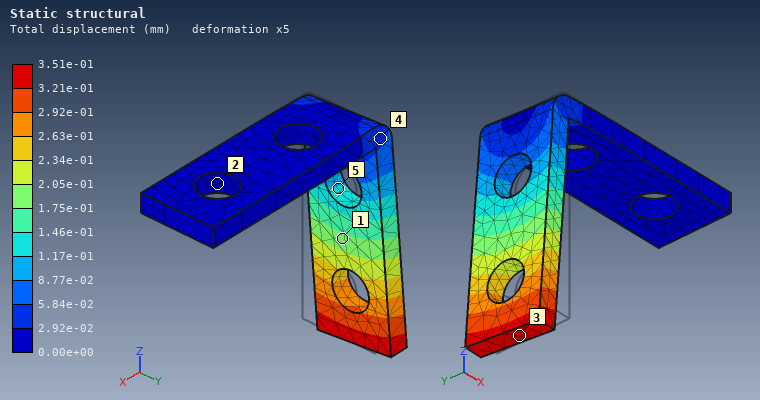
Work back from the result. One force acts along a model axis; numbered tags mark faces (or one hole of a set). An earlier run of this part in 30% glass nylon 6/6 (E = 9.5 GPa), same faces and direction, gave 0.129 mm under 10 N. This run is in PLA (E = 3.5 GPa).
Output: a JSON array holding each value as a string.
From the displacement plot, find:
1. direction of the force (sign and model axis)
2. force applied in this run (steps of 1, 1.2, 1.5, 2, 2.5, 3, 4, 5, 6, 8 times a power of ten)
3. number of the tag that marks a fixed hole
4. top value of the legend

["+Y", "10 N", "2", "3.51e-01 mm"]
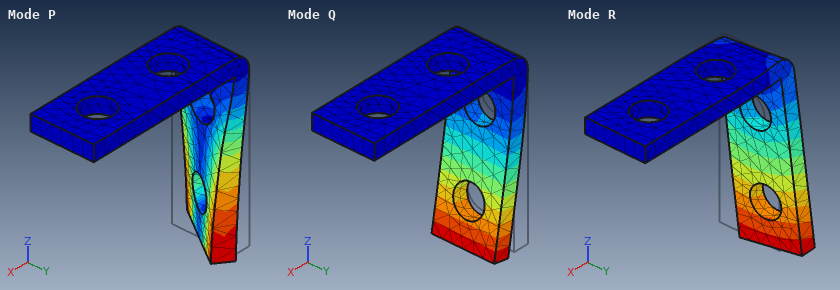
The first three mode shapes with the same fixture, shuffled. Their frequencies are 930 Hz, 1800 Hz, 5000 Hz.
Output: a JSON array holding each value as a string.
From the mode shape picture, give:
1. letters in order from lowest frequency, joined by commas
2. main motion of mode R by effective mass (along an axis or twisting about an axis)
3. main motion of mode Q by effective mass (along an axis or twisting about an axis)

["Q, R, P", "along Y", "along X"]
